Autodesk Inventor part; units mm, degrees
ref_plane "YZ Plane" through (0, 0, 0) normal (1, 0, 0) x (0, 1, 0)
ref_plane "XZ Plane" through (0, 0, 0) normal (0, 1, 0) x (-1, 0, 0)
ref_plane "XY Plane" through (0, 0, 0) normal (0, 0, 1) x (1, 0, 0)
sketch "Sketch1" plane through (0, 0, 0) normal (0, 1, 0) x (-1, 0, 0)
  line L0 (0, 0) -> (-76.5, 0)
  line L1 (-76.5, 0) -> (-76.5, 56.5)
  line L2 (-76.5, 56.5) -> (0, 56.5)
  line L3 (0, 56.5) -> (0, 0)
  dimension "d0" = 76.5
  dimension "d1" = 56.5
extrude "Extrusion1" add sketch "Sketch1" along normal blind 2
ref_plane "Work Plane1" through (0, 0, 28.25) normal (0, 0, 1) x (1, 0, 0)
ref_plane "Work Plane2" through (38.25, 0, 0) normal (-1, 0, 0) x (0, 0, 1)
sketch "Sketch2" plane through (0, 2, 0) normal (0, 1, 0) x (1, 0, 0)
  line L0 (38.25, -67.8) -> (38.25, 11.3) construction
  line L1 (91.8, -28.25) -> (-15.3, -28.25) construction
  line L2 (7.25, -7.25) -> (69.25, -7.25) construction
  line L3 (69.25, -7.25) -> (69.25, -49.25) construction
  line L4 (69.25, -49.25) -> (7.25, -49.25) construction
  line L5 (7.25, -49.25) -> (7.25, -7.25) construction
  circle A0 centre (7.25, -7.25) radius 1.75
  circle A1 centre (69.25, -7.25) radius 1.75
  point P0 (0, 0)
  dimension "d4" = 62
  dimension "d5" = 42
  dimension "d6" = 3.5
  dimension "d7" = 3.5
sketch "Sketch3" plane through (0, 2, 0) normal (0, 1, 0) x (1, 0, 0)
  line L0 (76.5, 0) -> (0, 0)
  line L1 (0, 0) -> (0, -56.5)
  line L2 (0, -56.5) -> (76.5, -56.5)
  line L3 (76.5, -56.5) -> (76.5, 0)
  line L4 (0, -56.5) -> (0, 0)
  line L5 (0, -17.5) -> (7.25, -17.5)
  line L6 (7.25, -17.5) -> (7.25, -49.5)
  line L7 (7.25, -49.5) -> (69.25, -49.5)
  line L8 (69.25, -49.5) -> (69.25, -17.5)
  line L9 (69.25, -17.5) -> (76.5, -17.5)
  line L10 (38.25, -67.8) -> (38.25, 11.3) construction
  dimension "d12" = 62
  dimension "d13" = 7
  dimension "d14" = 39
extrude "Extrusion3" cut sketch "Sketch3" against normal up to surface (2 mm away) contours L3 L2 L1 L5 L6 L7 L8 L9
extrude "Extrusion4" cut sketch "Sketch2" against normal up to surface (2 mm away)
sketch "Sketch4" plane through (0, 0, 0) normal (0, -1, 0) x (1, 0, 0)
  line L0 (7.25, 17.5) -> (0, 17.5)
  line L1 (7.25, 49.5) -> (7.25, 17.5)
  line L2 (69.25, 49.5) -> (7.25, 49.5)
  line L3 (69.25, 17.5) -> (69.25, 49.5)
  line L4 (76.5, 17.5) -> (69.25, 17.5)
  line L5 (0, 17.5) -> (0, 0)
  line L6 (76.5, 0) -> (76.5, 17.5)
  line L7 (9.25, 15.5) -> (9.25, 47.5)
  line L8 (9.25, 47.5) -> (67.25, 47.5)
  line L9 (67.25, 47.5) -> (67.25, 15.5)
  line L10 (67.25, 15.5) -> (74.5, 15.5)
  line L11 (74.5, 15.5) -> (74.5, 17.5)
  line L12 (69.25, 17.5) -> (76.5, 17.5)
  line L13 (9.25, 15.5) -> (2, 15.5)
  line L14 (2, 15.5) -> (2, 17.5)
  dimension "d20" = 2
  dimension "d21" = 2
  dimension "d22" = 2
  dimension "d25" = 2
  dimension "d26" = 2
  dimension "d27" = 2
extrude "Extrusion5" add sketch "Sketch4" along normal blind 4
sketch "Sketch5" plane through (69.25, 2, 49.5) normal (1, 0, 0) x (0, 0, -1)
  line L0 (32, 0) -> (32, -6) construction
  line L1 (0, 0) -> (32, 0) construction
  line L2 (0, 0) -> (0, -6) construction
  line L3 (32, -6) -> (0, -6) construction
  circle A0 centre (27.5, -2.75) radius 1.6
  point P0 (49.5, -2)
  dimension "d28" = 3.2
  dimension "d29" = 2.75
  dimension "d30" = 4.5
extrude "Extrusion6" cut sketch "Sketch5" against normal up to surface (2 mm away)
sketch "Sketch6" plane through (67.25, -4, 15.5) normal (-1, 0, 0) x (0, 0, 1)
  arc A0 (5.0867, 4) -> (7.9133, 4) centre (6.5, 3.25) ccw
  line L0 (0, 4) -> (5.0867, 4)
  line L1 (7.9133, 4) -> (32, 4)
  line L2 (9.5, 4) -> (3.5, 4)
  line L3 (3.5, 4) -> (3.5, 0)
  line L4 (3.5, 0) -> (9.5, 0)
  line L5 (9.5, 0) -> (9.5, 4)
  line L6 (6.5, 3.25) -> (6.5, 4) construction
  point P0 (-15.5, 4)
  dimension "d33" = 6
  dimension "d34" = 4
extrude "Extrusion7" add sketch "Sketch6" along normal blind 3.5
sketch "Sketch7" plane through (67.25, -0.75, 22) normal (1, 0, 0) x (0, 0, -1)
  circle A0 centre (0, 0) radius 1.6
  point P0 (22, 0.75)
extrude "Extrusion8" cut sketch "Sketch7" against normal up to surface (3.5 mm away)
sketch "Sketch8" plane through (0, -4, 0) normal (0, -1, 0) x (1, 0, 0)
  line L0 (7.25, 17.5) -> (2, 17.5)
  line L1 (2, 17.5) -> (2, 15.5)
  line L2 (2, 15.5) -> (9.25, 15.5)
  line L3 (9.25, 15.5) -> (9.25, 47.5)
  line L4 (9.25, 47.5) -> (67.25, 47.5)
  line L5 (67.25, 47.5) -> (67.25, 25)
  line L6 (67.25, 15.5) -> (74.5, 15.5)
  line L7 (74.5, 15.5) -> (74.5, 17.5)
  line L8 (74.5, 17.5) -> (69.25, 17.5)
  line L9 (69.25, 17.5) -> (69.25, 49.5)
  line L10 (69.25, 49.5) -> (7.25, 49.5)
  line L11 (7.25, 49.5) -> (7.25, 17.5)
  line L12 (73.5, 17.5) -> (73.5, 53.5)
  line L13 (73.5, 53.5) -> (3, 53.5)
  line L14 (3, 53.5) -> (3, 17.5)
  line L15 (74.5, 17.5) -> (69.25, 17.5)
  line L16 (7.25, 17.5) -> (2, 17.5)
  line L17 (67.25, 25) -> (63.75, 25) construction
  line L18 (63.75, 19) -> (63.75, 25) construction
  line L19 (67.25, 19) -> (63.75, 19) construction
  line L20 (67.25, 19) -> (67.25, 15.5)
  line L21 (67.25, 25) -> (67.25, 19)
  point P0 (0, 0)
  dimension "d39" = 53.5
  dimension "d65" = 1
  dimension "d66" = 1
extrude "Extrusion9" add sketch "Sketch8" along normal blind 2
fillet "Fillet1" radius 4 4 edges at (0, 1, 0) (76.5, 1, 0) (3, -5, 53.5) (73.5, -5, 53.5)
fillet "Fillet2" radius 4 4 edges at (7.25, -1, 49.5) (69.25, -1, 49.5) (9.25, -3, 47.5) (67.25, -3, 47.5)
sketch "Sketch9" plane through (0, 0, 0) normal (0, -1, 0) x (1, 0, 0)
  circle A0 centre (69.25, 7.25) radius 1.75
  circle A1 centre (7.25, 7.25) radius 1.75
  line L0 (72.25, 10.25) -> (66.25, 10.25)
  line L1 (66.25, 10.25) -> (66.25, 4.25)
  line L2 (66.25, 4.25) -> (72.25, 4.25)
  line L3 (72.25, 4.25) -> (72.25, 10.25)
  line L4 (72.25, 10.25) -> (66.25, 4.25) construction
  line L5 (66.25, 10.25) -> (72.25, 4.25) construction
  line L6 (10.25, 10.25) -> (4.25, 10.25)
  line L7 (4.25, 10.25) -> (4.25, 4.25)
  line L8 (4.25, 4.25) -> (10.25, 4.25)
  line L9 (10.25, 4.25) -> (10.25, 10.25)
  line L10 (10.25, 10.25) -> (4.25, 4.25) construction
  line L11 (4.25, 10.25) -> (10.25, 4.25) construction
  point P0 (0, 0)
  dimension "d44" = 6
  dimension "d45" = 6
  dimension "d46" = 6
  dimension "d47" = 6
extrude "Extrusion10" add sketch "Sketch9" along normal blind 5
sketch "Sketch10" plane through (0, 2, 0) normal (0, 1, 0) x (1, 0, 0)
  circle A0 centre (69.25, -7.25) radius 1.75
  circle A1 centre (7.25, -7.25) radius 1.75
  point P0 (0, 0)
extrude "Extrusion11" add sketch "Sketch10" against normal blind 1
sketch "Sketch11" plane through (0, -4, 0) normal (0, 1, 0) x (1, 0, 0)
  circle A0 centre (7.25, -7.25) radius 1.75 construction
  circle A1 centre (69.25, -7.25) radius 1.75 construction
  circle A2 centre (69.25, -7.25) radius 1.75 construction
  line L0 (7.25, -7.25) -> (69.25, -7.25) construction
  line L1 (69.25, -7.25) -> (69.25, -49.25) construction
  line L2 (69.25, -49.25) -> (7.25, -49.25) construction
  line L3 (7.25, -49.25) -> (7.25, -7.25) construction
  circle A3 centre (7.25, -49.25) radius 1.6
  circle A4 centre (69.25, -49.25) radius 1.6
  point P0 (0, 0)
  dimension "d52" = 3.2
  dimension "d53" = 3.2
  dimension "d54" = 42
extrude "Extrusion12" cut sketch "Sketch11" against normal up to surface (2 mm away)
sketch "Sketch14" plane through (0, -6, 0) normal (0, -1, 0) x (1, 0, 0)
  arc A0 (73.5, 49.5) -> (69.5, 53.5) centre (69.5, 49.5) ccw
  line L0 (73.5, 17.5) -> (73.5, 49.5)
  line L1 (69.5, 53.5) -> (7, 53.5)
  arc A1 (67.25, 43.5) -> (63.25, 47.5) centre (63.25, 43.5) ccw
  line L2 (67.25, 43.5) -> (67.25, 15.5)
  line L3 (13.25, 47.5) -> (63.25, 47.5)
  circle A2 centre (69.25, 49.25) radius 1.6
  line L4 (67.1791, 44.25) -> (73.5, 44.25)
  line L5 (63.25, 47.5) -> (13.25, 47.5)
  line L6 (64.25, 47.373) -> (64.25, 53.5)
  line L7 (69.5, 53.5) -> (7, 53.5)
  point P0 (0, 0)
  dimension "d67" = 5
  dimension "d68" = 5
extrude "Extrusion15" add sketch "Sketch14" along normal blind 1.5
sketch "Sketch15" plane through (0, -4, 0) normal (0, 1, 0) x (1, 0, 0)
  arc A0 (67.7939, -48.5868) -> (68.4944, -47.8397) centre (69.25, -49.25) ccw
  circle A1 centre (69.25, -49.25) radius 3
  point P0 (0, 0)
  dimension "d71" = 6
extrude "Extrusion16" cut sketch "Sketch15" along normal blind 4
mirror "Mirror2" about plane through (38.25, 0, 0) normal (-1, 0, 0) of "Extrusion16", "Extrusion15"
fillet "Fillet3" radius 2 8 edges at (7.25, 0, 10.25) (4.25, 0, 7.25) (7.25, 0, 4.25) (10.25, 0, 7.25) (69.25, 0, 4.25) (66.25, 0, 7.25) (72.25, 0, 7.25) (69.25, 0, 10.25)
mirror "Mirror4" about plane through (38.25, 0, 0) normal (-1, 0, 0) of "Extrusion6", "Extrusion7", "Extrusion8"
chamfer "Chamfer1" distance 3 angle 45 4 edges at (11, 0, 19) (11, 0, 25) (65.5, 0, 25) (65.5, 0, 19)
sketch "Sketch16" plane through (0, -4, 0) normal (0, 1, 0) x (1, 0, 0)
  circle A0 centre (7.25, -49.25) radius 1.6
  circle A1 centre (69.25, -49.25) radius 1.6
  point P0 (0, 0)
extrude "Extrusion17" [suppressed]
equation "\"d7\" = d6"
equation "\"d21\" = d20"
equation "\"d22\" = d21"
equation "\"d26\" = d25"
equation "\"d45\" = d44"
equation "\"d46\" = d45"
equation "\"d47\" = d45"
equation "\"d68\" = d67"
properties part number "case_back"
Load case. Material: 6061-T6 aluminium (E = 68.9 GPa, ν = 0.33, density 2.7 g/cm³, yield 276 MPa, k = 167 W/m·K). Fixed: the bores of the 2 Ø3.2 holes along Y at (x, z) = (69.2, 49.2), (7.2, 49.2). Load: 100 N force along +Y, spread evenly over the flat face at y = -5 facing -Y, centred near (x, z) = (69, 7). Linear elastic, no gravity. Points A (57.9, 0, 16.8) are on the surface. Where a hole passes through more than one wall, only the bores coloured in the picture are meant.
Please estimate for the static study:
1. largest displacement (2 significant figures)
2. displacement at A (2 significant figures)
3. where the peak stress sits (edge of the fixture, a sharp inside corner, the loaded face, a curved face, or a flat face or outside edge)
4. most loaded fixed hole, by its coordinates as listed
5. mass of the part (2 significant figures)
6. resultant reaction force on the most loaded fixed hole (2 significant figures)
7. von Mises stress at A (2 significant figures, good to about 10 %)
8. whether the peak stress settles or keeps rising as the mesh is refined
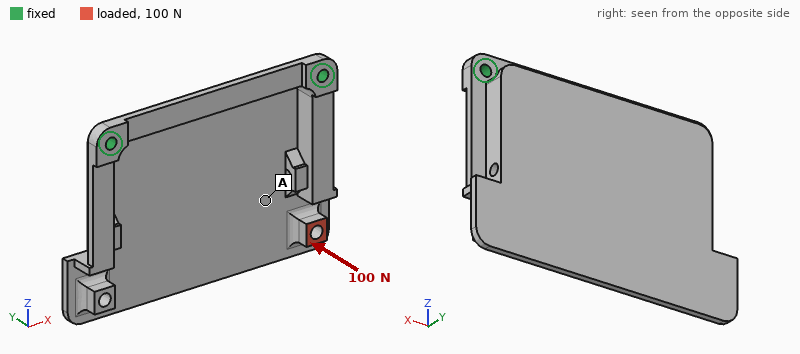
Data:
0.49 mm
0.23 mm
edge of the fixture
(69.2, 49.2)
27 g
120 N
17 MPa
keeps rising
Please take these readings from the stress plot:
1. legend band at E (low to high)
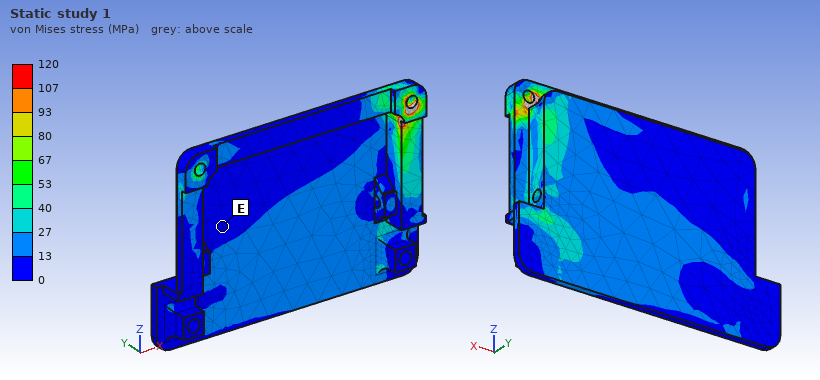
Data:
0 to 13 MPa
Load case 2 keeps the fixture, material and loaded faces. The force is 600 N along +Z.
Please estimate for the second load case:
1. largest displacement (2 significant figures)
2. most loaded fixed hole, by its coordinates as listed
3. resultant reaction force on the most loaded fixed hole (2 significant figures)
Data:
0.38 mm
(69.2, 49.2)
600 N
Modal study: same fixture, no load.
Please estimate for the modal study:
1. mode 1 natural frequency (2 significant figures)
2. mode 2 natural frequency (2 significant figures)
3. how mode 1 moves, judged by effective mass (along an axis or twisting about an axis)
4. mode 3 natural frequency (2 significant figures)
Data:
1000 Hz
1600 Hz
along Y
3100 Hz
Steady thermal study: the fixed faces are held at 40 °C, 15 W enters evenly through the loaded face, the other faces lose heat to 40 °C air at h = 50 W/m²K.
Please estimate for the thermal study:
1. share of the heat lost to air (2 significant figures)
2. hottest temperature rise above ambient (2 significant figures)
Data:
43 %
60 K
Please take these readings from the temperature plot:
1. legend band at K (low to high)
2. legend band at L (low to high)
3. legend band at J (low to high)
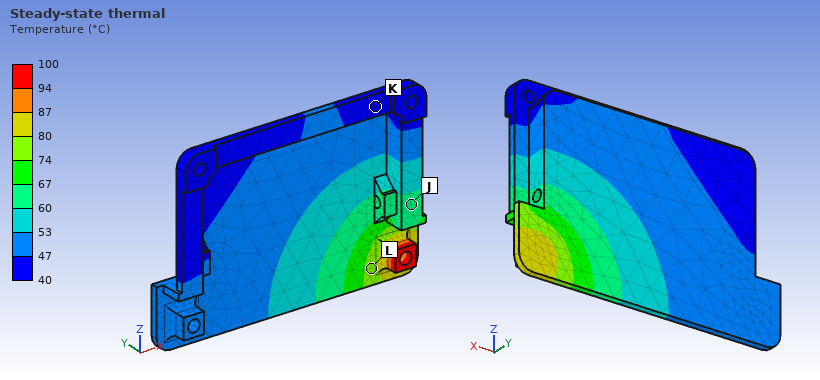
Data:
40 to 47 °C
74 to 80 °C
60 to 67 °C
